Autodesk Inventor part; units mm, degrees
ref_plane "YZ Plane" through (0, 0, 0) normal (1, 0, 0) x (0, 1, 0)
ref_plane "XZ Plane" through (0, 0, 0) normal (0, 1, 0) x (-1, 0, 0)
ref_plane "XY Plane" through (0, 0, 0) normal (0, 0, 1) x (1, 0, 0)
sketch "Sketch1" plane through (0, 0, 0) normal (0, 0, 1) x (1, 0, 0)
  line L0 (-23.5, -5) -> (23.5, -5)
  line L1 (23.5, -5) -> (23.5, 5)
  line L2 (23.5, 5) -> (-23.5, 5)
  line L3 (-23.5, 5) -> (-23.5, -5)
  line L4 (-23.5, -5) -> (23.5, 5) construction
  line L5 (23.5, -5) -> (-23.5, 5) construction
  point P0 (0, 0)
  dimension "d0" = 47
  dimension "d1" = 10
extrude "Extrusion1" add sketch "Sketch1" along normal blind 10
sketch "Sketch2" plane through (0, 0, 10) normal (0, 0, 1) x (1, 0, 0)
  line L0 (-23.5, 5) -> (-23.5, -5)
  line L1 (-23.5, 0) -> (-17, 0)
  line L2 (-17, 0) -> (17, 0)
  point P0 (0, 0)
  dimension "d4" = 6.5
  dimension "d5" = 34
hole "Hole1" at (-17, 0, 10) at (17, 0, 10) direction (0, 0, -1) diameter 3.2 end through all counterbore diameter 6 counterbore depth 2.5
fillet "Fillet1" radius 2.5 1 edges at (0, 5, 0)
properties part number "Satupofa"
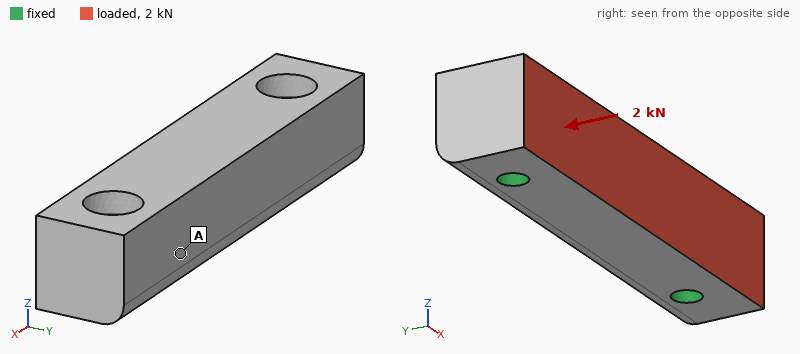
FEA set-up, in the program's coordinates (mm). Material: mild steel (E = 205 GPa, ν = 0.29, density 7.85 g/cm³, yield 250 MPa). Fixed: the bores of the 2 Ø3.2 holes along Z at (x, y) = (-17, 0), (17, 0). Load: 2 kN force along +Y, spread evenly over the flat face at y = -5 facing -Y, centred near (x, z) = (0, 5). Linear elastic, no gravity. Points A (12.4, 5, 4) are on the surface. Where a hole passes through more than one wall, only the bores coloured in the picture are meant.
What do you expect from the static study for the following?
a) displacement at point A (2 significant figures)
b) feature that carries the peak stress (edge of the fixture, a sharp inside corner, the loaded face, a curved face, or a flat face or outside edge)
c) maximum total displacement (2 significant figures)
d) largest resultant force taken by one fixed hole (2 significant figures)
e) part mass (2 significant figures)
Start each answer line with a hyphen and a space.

- 1.1 µm
- edge of the fixture
- 2.8 µm
- 1.0 kN
- 34 g
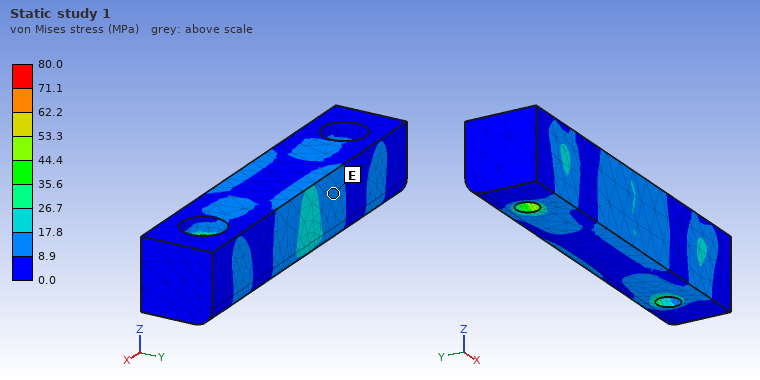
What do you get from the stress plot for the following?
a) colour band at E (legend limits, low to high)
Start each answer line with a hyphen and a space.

- 8.9 to 17.8 MPa
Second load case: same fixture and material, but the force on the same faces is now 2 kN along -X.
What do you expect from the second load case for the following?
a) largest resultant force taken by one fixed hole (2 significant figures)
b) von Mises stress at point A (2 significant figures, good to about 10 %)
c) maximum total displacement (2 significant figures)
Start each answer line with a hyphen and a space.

- 1.0 kN
- 5.8 MPa
- 1.1 µm
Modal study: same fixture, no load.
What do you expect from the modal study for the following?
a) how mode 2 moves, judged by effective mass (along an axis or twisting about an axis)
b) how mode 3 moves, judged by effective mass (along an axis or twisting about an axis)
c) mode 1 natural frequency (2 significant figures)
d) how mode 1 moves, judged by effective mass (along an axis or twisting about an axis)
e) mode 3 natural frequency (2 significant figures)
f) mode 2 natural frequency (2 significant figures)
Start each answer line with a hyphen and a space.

- along Z
- twisting about X
- 25 kHz
- along Y
- 39 kHz
- 28 kHz
